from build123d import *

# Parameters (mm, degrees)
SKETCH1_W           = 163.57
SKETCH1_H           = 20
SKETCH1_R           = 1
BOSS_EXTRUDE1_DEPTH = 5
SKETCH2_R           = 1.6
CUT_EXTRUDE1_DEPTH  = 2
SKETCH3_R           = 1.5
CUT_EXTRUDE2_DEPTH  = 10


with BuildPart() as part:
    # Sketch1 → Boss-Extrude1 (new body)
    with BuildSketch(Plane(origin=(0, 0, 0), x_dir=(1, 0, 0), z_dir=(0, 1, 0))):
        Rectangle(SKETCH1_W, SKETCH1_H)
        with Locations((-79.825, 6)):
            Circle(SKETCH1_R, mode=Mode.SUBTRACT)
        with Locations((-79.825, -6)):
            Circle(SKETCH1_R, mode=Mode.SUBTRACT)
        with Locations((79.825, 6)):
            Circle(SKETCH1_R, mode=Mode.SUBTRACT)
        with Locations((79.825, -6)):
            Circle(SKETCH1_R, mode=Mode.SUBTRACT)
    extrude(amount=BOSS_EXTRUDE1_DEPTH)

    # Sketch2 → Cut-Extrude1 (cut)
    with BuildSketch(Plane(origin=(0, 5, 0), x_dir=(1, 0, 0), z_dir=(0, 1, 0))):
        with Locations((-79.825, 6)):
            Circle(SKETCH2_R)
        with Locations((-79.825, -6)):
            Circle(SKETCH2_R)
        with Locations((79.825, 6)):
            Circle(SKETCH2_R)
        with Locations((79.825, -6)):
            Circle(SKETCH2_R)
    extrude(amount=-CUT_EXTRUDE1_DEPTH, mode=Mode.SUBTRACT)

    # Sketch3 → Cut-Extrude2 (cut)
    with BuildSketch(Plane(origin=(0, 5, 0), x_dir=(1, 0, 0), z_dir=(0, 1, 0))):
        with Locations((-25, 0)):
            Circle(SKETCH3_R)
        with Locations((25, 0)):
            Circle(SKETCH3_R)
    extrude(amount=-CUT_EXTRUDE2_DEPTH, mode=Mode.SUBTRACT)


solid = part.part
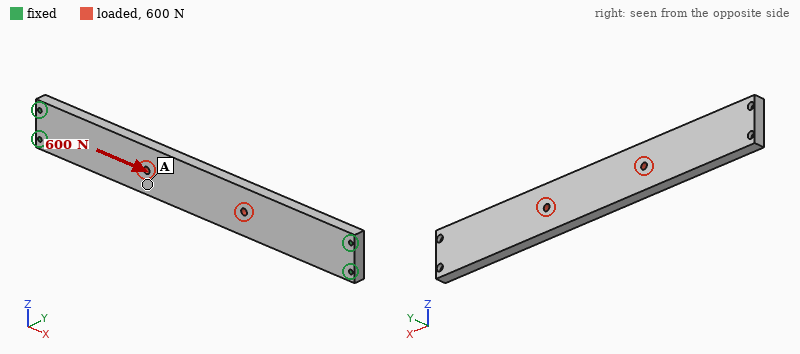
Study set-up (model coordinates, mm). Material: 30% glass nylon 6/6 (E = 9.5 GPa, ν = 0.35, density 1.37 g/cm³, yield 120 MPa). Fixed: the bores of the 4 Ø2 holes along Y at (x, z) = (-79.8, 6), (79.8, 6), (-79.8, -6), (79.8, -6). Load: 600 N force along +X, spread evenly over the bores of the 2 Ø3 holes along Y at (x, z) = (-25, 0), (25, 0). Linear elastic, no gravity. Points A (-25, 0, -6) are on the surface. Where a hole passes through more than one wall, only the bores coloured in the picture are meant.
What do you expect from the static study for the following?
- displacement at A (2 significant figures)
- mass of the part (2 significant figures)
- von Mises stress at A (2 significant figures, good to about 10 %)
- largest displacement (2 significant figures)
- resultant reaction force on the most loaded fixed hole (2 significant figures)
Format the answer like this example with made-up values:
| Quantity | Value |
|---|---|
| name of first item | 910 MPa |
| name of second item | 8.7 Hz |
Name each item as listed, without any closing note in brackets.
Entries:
| Quantity | Value |
|---|---|
| displacement at A | 23 µm |
| mass of the part | 22 g |
| von Mises stress at A | 1.8 MPa |
| largest displacement | 26 µm |
| resultant reaction force on the most loaded fixed hole | 150 N |
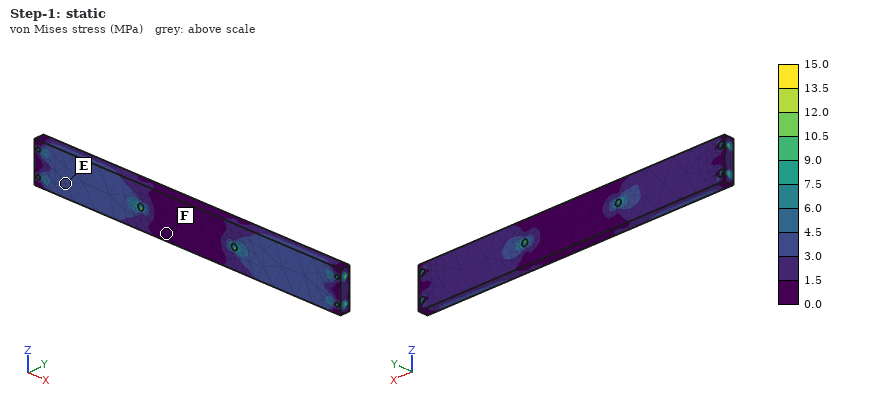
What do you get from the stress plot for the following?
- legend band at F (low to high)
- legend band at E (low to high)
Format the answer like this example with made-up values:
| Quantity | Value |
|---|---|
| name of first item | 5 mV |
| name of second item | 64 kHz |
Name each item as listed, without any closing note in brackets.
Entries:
| Quantity | Value |
|---|---|
| legend band at F | 0.0 to 1.5 MPa |
| legend band at E | 3.0 to 4.5 MPa |
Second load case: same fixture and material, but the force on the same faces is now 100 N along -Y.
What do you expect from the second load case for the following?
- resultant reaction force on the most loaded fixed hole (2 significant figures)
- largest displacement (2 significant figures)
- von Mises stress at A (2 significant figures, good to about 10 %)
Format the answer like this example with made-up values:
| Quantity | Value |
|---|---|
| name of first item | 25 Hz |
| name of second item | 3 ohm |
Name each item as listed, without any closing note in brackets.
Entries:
| Quantity | Value |
|---|---|
| resultant reaction force on the most loaded fixed hole | 48 N |
| largest displacement | 1.1 mm |
| von Mises stress at A | 13 MPa |
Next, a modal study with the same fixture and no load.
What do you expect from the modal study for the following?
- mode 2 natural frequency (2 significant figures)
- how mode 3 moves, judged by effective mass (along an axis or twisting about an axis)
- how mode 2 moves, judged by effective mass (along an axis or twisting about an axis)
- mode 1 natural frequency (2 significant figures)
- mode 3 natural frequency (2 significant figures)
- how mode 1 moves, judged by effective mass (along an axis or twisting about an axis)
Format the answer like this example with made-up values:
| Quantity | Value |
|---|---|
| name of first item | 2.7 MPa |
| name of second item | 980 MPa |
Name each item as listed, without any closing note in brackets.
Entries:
| Quantity | Value |
|---|---|
| mode 2 natural frequency | 1300 Hz |
| how mode 3 moves, judged by effective mass | along Z |
| how mode 2 moves, judged by effective mass | twisting about Z |
| mode 1 natural frequency | 460 Hz |
| mode 3 natural frequency | 1700 Hz |
| how mode 1 moves, judged by effective mass | along Y |
